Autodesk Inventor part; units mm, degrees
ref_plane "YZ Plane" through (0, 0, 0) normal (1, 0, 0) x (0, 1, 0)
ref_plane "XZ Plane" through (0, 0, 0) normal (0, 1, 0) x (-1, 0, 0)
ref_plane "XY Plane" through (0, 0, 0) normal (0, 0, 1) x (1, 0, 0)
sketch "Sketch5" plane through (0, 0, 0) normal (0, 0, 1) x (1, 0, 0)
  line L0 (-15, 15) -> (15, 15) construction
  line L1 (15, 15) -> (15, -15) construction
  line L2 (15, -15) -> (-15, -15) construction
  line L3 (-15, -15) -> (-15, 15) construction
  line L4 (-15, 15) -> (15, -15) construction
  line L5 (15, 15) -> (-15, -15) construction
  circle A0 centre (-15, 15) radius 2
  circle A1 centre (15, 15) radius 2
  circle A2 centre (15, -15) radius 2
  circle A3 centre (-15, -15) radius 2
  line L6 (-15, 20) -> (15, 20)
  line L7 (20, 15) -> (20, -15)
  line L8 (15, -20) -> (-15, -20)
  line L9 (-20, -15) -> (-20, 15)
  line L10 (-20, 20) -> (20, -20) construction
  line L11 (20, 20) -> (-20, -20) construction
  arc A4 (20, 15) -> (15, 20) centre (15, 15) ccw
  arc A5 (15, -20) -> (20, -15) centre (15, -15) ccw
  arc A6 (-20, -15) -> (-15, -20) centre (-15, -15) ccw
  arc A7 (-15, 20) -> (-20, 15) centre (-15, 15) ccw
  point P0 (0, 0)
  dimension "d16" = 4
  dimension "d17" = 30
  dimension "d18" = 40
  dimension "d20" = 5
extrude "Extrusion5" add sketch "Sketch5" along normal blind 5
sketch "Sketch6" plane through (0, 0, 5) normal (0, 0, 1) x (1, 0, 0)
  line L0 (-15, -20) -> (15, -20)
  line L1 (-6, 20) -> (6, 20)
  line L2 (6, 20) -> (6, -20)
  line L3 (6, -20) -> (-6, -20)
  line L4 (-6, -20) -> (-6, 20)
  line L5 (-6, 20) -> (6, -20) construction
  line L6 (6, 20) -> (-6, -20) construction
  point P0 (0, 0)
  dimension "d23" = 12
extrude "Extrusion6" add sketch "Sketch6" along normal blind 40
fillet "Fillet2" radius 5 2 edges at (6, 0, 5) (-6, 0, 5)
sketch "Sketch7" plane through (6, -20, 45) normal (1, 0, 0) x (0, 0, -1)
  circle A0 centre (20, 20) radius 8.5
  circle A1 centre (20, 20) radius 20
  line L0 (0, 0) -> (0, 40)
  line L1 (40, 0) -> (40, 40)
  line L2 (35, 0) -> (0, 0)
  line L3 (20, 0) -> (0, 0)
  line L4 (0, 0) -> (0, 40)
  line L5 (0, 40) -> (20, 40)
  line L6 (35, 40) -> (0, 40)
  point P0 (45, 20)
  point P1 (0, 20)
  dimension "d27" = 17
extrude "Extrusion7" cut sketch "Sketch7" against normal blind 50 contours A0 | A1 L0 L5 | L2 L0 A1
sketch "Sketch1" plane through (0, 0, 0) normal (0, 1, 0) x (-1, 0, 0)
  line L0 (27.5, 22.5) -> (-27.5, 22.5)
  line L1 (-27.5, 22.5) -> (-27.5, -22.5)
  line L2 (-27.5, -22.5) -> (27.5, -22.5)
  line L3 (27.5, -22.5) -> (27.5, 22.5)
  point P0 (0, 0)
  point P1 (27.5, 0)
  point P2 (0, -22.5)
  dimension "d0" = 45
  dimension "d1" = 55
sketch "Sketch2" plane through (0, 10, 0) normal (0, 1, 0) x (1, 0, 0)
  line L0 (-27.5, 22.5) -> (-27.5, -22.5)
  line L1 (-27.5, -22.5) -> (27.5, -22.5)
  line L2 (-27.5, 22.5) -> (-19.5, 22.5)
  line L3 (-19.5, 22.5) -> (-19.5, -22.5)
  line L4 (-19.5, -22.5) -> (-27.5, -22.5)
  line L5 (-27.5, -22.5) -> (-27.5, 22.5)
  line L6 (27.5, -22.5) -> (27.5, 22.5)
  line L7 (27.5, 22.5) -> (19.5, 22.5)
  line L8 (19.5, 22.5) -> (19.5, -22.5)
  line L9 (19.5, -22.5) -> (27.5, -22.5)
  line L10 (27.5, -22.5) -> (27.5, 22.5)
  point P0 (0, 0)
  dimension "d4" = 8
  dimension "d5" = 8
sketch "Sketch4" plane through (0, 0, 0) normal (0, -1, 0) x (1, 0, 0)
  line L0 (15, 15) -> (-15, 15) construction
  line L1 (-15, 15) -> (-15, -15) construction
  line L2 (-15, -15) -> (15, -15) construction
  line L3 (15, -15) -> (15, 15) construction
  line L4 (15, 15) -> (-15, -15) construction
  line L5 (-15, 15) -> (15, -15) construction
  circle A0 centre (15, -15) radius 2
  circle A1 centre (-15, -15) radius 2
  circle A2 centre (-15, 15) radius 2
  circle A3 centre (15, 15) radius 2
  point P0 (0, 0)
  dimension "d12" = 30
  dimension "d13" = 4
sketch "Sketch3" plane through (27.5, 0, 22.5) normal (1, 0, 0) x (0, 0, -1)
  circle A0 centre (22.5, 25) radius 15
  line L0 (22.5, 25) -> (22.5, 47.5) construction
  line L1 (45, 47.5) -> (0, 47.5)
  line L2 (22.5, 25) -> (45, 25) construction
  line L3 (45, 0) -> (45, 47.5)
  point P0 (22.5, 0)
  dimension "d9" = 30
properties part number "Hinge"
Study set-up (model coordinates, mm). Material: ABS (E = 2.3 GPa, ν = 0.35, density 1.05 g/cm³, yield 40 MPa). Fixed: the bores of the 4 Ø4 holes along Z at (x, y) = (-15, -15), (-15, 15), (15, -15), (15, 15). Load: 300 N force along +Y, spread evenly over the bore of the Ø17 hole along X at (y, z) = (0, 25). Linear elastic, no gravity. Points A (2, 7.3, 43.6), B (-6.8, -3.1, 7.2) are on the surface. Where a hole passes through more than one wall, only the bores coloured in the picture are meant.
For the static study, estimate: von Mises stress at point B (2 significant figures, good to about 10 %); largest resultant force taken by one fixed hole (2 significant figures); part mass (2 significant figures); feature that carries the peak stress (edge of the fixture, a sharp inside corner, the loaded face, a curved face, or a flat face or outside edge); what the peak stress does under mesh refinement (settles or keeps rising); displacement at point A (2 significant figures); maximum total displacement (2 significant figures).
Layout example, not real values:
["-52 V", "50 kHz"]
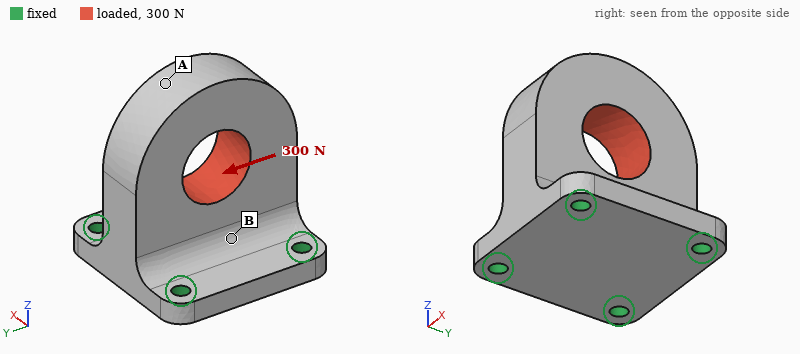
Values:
["3.0 MPa", "150 N", "24 g", "edge of the fixture", "keeps rising", "0.17 mm", "0.17 mm"]
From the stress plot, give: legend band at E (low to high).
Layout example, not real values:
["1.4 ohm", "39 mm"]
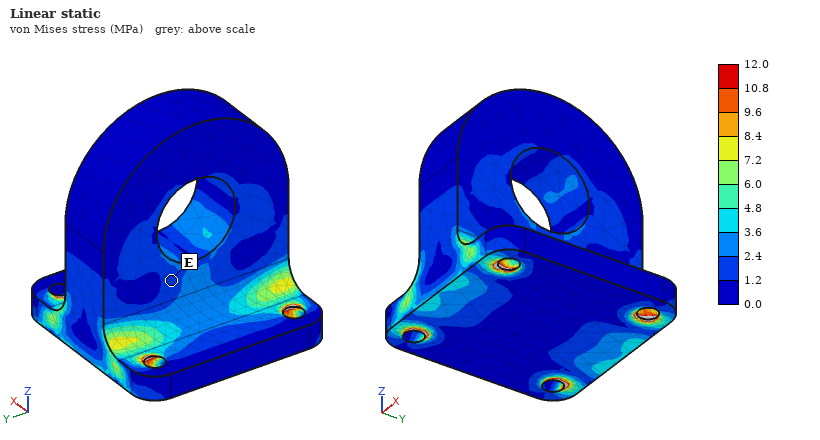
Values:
["1.2 to 2.4 MPa"]
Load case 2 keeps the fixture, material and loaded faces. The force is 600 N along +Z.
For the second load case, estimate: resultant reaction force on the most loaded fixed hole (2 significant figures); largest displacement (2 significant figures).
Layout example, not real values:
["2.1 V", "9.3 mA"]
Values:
["160 N", "76 µm"]
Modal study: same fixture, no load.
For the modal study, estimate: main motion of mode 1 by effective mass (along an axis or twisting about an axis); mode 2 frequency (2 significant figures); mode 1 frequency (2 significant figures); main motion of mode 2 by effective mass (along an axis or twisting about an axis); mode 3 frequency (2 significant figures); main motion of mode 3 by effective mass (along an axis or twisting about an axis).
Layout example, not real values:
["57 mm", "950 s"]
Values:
["along X", "2000 Hz", "1500 Hz", "along Y", "3700 Hz", "twisting about Z"]
